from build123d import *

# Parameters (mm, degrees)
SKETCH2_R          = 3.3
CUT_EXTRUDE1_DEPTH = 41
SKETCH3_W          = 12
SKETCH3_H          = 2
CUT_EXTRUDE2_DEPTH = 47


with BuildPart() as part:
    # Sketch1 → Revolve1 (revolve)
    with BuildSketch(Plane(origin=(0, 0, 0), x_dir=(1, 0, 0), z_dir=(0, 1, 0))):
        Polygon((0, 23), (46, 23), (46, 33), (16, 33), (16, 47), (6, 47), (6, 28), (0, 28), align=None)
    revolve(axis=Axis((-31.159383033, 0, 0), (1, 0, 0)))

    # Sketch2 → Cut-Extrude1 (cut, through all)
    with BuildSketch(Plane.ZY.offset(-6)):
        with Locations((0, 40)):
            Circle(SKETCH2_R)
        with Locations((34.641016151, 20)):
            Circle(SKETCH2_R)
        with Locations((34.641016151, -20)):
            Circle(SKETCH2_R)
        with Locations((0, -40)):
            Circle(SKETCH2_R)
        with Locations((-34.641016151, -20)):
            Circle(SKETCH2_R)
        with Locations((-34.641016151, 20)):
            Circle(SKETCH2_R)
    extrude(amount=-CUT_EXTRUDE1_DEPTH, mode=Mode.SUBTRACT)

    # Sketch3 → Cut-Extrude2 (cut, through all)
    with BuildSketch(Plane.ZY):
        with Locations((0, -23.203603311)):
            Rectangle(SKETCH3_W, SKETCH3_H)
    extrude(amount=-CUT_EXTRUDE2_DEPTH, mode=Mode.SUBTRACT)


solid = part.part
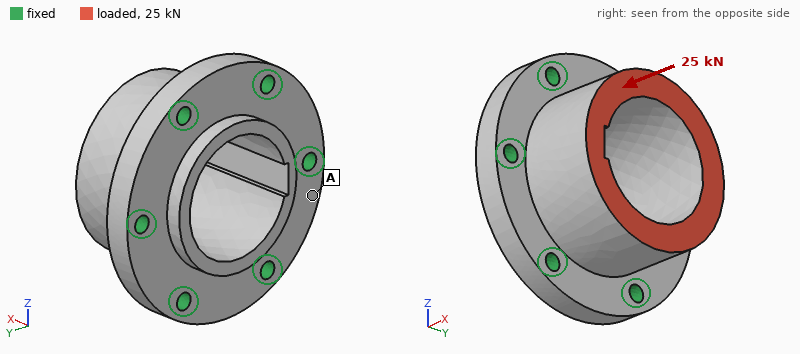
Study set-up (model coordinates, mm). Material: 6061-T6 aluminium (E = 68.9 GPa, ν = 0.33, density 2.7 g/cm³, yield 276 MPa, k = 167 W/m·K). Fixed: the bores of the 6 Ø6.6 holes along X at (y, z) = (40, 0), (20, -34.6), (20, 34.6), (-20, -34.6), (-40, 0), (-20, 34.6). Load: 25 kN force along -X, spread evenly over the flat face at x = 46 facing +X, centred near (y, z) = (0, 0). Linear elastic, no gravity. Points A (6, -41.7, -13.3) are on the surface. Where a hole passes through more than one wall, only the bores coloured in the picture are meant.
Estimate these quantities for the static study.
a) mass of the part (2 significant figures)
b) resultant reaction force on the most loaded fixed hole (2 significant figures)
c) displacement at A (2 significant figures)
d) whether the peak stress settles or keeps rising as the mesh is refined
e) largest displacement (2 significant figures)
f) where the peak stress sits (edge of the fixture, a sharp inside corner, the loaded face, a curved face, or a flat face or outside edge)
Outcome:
290 g
4.4 kN
4.1 µm
keeps rising
18 µm
edge of the fixture
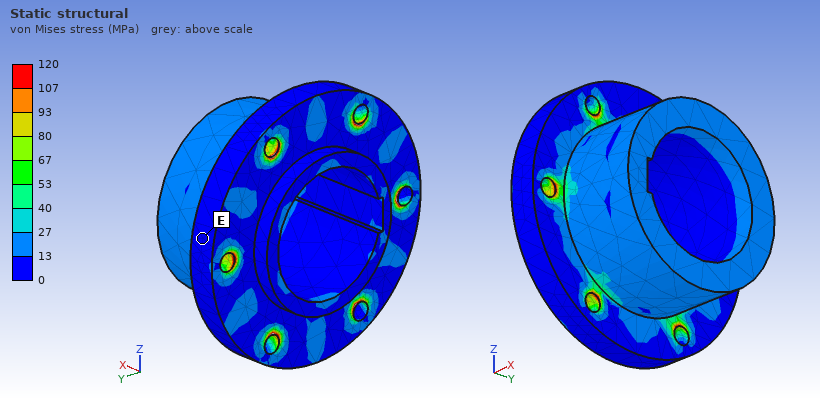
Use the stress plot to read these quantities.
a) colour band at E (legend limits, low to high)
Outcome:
0 to 13 MPa
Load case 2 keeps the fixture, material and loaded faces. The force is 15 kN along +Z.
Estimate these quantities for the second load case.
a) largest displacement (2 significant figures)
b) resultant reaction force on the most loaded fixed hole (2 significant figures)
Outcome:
51 µm
4.9 kN
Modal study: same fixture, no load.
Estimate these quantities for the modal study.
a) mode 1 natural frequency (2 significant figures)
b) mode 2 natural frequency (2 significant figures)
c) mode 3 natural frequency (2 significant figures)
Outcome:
12 kHz
13 kHz
13 kHz
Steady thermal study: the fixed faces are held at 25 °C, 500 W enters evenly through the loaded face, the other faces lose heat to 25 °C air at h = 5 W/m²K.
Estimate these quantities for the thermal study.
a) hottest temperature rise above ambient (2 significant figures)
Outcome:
75 K
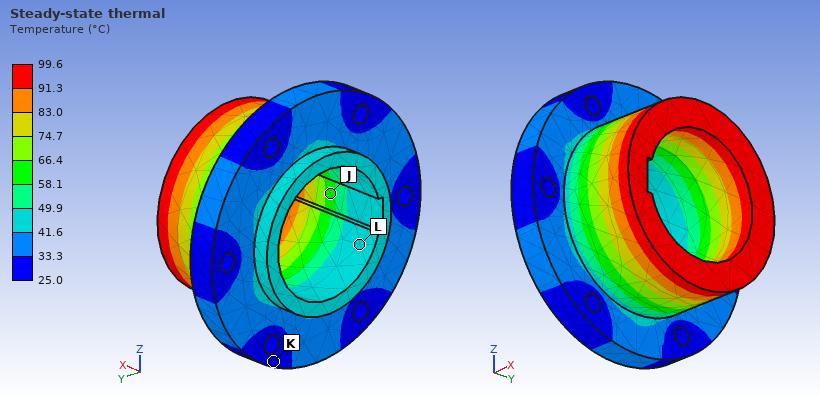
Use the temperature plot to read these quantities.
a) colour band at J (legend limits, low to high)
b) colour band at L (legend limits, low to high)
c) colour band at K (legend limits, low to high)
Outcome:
58.1 to 66.4 °C
41.6 to 49.9 °C
25.0 to 33.3 °C
